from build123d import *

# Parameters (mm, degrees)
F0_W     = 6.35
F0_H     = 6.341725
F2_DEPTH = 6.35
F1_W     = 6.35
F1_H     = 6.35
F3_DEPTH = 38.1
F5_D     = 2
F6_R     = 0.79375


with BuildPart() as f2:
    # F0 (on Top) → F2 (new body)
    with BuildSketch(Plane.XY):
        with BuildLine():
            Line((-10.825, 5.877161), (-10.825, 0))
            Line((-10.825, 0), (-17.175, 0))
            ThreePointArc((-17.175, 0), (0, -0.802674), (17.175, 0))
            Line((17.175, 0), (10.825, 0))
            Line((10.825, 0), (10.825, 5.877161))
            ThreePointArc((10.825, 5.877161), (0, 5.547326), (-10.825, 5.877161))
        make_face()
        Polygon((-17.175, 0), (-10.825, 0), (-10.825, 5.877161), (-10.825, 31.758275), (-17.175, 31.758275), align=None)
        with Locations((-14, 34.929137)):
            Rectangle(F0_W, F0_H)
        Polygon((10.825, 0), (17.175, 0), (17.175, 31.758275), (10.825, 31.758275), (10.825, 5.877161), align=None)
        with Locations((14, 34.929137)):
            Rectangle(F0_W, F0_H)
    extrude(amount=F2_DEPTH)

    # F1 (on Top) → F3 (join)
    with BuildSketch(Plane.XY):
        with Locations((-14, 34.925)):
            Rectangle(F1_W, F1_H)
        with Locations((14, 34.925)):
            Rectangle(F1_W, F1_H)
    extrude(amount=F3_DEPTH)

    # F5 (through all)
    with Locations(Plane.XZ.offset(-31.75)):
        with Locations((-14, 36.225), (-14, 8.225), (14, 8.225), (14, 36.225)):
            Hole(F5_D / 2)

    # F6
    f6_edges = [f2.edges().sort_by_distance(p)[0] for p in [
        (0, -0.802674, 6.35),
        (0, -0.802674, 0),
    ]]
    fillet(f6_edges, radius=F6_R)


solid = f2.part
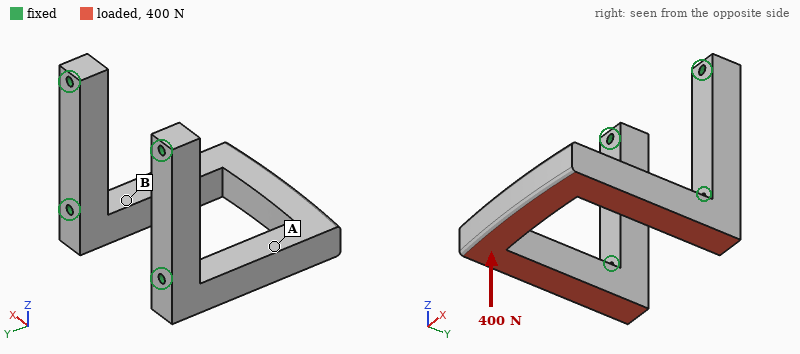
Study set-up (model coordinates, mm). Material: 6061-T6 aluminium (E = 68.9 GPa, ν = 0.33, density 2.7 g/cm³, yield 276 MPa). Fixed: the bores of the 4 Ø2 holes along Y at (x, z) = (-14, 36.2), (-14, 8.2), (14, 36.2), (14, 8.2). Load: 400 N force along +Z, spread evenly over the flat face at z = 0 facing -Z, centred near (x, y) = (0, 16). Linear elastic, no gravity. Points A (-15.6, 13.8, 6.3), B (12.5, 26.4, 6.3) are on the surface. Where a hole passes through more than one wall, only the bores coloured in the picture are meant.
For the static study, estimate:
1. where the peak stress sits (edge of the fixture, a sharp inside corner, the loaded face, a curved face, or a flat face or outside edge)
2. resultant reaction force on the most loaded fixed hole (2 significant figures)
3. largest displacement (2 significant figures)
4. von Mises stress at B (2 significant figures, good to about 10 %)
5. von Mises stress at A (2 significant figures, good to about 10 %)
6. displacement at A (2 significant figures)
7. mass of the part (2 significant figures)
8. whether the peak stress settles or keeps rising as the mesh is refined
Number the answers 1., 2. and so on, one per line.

1. a sharp inside corner
2. 200 N
3. 0.19 mm
4. 54 MPa
5. 19 MPa
6. 0.092 mm
7. 17 g
8. keeps rising
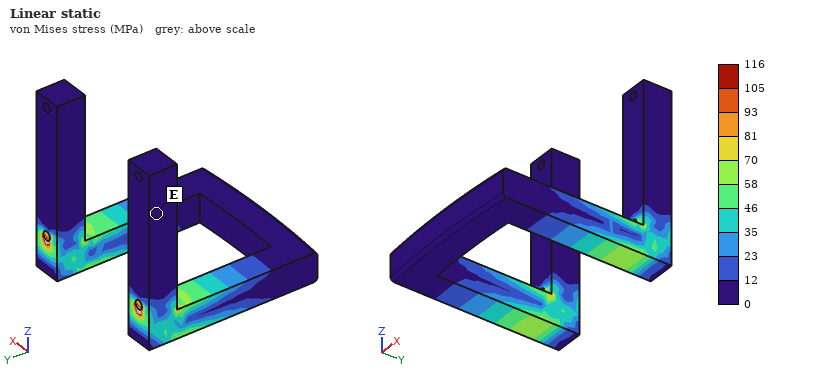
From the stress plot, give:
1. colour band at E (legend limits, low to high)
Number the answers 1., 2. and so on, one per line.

1. 0 to 12 MPa
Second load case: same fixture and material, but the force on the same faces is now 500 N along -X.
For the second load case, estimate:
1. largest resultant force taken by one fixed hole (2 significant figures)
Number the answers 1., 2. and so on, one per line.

1. 310 N
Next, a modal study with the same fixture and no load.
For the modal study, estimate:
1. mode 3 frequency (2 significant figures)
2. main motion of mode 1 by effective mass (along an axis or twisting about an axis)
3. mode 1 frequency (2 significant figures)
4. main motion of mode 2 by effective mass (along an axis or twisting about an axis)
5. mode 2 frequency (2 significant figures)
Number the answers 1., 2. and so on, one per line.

1. 5500 Hz
2. along Z
3. 2500 Hz
4. along X
5. 4100 Hz
